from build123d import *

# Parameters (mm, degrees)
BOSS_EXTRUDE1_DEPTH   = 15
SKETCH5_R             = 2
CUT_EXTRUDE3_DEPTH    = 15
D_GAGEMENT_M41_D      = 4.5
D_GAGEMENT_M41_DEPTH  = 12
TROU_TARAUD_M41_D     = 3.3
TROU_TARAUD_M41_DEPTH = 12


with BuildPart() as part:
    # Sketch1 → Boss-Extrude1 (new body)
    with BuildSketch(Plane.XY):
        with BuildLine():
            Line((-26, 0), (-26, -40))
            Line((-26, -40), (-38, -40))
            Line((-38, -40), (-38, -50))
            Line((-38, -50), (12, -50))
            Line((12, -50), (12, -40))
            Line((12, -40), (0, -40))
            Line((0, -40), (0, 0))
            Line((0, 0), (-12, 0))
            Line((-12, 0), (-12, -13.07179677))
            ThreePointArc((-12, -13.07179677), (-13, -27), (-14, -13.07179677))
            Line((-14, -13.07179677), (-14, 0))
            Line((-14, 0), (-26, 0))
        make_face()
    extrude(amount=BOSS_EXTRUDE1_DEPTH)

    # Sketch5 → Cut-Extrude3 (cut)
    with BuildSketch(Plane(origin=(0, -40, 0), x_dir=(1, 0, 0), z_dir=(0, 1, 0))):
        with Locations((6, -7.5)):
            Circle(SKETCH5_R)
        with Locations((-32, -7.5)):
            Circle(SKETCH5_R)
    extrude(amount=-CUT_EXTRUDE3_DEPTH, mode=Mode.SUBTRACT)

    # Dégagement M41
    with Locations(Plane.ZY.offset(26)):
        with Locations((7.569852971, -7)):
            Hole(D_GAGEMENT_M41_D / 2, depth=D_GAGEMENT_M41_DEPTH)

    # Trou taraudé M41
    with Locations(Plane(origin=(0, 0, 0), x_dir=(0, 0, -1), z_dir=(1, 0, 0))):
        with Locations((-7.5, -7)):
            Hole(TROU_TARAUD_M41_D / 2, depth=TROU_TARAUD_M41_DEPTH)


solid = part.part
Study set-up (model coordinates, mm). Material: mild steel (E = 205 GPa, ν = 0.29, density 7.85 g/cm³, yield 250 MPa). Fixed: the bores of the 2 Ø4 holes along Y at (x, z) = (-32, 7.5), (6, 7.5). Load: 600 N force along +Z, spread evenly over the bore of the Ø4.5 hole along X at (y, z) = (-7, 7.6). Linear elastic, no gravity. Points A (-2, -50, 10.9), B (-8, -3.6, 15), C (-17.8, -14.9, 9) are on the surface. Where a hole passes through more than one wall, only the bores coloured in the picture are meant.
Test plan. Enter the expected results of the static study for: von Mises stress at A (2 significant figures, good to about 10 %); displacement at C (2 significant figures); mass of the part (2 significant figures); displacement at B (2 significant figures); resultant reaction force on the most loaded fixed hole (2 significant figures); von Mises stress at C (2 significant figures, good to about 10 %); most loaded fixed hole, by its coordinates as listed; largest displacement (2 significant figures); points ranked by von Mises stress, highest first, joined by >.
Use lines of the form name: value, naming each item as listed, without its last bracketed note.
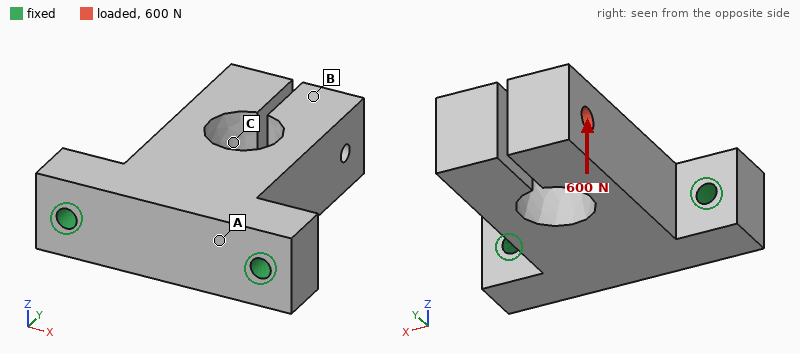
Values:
von Mises stress at A: 24 MPa
displacement at C: 25 µm
mass of the part: 160 g
displacement at B: 21 µm
resultant reaction force on the most loaded fixed hole: 410 N
von Mises stress at C: 13 MPa
most loaded fixed hole, by its coordinates as listed: (-32, 7.5)
largest displacement: 43 µm
points ranked by von Mises stress, highest first, joined by >: A > C > B
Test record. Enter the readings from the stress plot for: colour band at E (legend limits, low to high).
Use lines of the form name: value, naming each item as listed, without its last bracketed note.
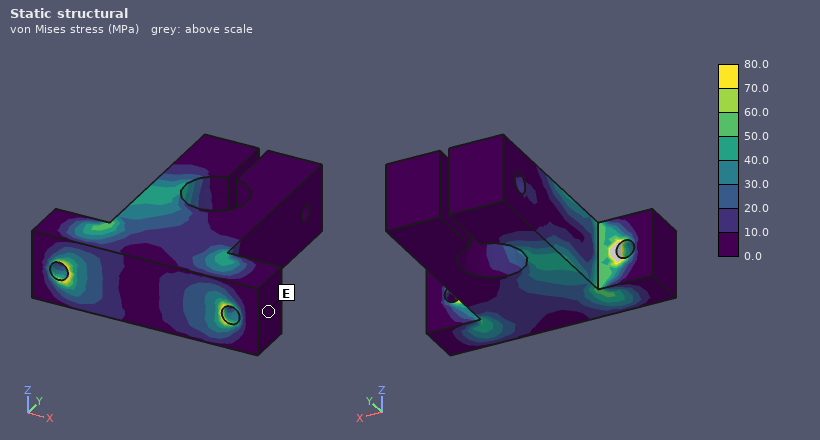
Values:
colour band at E: 0.0 to 10.0 MPa
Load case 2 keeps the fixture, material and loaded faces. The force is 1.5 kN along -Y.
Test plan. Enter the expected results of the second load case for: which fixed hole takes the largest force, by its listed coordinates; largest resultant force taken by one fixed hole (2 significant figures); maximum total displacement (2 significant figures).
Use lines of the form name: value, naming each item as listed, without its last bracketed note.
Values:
which fixed hole takes the largest force, by its listed coordinates: (-32, 7.5)
largest resultant force taken by one fixed hole: 1.1 kN
maximum total displacement: 17 µm
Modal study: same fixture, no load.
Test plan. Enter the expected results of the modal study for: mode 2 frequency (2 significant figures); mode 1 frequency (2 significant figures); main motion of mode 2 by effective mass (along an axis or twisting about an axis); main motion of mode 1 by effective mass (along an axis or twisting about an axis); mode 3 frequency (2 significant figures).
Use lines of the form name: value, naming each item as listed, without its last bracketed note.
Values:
mode 2 frequency: 4600 Hz
mode 1 frequency: 3500 Hz
main motion of mode 2 by effective mass: along X
main motion of mode 1 by effective mass: along Z
mode 3 frequency: 4900 Hz
